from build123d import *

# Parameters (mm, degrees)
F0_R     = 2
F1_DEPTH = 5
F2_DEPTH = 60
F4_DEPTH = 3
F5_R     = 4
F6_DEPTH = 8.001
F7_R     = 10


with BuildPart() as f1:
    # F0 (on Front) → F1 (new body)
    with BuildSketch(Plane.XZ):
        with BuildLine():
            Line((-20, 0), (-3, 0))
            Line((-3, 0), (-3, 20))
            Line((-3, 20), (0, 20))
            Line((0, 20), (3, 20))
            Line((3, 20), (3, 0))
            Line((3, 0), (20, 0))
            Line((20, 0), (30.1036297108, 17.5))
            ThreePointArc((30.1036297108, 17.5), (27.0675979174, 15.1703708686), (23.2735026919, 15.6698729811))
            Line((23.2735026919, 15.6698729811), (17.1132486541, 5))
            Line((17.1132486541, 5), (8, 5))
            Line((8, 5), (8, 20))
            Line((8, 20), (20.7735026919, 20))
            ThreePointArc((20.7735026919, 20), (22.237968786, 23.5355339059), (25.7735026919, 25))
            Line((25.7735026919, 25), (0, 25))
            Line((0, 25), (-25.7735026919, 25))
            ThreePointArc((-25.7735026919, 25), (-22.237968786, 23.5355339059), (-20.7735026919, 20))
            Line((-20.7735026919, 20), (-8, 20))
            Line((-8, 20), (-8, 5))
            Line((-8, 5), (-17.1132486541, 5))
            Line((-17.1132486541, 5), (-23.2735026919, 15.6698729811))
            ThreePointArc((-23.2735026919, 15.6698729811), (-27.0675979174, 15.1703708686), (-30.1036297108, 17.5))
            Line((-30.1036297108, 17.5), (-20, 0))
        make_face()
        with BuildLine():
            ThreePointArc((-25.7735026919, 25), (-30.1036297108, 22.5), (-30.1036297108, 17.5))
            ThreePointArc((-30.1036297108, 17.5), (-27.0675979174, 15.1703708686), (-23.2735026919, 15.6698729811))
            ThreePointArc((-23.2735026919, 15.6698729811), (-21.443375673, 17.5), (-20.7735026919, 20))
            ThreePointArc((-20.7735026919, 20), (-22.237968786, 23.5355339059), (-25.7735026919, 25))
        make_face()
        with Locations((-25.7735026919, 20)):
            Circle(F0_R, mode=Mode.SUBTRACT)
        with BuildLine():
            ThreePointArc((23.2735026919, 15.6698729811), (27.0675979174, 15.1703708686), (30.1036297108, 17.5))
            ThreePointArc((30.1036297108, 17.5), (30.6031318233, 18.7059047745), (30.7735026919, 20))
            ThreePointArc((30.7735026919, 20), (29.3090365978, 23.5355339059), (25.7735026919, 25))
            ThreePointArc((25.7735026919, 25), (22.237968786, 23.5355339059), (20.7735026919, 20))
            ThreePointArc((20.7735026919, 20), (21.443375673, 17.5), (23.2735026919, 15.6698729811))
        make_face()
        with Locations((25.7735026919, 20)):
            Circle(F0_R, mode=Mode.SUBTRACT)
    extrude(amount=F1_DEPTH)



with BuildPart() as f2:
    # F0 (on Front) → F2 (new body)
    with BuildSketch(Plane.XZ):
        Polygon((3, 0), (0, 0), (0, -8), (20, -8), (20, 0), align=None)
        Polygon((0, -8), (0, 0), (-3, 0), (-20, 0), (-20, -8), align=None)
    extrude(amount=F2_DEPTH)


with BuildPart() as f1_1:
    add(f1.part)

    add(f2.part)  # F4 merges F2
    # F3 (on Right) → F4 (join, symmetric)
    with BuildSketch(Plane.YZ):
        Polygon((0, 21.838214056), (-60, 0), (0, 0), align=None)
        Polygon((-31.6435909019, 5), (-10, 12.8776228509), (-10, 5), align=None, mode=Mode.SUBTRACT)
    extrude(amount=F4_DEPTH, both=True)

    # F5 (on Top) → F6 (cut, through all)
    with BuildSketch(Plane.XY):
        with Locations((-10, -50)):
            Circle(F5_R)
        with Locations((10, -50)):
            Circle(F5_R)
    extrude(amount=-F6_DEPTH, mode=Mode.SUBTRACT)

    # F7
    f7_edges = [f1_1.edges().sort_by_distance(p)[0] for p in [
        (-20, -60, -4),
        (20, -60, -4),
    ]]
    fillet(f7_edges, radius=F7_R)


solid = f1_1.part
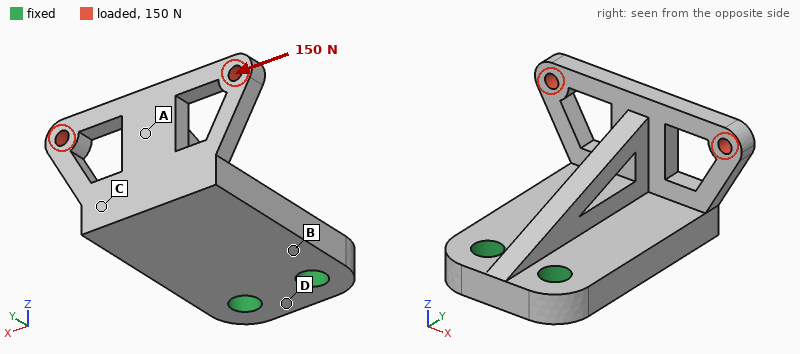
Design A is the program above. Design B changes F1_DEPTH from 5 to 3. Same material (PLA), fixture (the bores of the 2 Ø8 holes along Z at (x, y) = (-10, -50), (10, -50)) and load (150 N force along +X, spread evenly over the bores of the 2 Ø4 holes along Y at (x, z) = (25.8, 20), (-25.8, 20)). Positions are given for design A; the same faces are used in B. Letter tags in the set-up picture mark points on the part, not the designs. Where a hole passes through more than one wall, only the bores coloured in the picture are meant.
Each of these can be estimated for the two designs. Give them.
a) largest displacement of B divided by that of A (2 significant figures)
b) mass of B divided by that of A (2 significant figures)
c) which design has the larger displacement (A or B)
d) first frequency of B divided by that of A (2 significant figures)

1.2
0.94
B
1.1
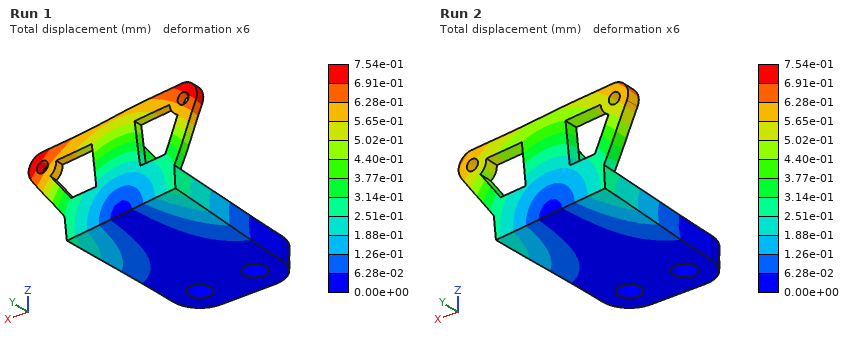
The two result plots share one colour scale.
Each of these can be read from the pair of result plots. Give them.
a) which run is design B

Run 1
